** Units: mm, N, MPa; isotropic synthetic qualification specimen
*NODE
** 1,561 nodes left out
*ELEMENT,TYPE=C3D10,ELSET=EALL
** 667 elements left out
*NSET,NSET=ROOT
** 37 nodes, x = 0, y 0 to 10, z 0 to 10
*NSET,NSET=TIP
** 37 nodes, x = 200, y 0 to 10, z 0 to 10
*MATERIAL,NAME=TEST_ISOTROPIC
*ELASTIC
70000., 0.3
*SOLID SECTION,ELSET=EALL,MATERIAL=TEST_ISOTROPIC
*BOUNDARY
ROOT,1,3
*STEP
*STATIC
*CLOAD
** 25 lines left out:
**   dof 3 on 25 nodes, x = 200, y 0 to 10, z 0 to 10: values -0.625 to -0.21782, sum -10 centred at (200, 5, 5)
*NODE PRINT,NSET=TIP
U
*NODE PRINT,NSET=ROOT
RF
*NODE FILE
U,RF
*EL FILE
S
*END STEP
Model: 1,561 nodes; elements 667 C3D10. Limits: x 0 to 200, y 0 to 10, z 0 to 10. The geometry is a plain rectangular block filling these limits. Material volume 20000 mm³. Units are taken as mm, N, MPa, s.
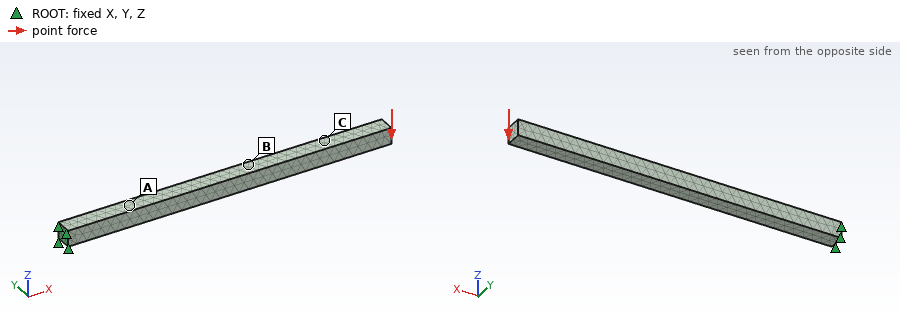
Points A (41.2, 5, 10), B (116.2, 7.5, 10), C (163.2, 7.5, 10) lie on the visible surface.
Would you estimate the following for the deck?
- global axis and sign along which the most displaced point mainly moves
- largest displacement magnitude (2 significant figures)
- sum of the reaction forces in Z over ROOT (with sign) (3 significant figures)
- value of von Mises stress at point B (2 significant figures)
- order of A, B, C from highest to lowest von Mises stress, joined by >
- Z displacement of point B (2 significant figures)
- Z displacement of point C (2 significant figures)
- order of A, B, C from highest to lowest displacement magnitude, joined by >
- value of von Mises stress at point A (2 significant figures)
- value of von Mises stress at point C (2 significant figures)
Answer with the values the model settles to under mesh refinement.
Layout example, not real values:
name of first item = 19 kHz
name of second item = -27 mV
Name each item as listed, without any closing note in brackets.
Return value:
global axis and sign along which the most displaced point mainly moves = -Z
largest displacement magnitude = 0.46 mm
sum of the reaction forces in Z over ROOT (with sign) = 10.0 N
value of von Mises stress at point B = 5.0 MPa
order of A, B, C from highest to lowest von Mises stress, joined by > = A > B > C
Z displacement of point B = -0.19 mm
Z displacement of point C = -0.33 mm
order of A, B, C from highest to lowest displacement magnitude, joined by > = C > B > A
value of von Mises stress at point A = 9.5 MPa
value of von Mises stress at point C = 2.2 MPa
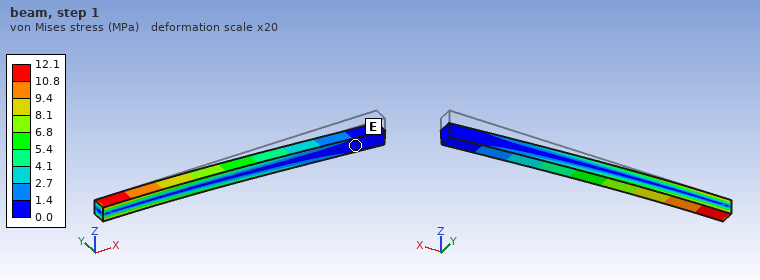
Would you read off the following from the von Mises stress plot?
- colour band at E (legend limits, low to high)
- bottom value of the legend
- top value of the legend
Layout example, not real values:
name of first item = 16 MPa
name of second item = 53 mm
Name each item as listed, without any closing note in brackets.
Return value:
colour band at E = 0.0 to 1.4 MPa
bottom value of the legend = 0.0 MPa
top value of the legend = 12.1 MPa
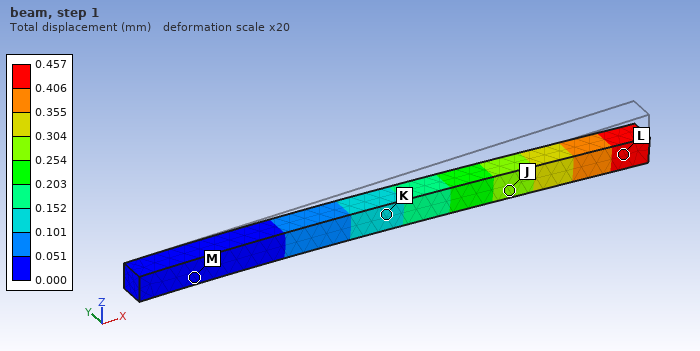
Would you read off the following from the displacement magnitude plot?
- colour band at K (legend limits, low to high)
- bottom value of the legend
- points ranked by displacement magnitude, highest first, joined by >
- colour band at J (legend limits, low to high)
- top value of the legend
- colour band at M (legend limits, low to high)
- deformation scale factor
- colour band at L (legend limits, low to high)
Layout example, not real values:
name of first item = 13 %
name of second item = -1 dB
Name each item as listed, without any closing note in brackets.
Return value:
colour band at K = 0.101 to 0.152 mm
bottom value of the legend = 0.000 mm
points ranked by displacement magnitude, highest first, joined by > = L > J > K > M
colour band at J = 0.254 to 0.304 mm
top value of the legend = 0.457 mm
colour band at M = 0.000 to 0.051 mm
deformation scale factor = 20
colour band at L = 0.406 to 0.457 mm
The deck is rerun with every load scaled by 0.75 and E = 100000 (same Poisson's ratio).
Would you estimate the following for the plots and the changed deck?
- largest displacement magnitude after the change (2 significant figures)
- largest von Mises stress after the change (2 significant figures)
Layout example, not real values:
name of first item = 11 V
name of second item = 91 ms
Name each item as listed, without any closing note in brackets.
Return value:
largest displacement magnitude after the change = 0.24 mm
largest von Mises stress after the change = 9.1 MPa
